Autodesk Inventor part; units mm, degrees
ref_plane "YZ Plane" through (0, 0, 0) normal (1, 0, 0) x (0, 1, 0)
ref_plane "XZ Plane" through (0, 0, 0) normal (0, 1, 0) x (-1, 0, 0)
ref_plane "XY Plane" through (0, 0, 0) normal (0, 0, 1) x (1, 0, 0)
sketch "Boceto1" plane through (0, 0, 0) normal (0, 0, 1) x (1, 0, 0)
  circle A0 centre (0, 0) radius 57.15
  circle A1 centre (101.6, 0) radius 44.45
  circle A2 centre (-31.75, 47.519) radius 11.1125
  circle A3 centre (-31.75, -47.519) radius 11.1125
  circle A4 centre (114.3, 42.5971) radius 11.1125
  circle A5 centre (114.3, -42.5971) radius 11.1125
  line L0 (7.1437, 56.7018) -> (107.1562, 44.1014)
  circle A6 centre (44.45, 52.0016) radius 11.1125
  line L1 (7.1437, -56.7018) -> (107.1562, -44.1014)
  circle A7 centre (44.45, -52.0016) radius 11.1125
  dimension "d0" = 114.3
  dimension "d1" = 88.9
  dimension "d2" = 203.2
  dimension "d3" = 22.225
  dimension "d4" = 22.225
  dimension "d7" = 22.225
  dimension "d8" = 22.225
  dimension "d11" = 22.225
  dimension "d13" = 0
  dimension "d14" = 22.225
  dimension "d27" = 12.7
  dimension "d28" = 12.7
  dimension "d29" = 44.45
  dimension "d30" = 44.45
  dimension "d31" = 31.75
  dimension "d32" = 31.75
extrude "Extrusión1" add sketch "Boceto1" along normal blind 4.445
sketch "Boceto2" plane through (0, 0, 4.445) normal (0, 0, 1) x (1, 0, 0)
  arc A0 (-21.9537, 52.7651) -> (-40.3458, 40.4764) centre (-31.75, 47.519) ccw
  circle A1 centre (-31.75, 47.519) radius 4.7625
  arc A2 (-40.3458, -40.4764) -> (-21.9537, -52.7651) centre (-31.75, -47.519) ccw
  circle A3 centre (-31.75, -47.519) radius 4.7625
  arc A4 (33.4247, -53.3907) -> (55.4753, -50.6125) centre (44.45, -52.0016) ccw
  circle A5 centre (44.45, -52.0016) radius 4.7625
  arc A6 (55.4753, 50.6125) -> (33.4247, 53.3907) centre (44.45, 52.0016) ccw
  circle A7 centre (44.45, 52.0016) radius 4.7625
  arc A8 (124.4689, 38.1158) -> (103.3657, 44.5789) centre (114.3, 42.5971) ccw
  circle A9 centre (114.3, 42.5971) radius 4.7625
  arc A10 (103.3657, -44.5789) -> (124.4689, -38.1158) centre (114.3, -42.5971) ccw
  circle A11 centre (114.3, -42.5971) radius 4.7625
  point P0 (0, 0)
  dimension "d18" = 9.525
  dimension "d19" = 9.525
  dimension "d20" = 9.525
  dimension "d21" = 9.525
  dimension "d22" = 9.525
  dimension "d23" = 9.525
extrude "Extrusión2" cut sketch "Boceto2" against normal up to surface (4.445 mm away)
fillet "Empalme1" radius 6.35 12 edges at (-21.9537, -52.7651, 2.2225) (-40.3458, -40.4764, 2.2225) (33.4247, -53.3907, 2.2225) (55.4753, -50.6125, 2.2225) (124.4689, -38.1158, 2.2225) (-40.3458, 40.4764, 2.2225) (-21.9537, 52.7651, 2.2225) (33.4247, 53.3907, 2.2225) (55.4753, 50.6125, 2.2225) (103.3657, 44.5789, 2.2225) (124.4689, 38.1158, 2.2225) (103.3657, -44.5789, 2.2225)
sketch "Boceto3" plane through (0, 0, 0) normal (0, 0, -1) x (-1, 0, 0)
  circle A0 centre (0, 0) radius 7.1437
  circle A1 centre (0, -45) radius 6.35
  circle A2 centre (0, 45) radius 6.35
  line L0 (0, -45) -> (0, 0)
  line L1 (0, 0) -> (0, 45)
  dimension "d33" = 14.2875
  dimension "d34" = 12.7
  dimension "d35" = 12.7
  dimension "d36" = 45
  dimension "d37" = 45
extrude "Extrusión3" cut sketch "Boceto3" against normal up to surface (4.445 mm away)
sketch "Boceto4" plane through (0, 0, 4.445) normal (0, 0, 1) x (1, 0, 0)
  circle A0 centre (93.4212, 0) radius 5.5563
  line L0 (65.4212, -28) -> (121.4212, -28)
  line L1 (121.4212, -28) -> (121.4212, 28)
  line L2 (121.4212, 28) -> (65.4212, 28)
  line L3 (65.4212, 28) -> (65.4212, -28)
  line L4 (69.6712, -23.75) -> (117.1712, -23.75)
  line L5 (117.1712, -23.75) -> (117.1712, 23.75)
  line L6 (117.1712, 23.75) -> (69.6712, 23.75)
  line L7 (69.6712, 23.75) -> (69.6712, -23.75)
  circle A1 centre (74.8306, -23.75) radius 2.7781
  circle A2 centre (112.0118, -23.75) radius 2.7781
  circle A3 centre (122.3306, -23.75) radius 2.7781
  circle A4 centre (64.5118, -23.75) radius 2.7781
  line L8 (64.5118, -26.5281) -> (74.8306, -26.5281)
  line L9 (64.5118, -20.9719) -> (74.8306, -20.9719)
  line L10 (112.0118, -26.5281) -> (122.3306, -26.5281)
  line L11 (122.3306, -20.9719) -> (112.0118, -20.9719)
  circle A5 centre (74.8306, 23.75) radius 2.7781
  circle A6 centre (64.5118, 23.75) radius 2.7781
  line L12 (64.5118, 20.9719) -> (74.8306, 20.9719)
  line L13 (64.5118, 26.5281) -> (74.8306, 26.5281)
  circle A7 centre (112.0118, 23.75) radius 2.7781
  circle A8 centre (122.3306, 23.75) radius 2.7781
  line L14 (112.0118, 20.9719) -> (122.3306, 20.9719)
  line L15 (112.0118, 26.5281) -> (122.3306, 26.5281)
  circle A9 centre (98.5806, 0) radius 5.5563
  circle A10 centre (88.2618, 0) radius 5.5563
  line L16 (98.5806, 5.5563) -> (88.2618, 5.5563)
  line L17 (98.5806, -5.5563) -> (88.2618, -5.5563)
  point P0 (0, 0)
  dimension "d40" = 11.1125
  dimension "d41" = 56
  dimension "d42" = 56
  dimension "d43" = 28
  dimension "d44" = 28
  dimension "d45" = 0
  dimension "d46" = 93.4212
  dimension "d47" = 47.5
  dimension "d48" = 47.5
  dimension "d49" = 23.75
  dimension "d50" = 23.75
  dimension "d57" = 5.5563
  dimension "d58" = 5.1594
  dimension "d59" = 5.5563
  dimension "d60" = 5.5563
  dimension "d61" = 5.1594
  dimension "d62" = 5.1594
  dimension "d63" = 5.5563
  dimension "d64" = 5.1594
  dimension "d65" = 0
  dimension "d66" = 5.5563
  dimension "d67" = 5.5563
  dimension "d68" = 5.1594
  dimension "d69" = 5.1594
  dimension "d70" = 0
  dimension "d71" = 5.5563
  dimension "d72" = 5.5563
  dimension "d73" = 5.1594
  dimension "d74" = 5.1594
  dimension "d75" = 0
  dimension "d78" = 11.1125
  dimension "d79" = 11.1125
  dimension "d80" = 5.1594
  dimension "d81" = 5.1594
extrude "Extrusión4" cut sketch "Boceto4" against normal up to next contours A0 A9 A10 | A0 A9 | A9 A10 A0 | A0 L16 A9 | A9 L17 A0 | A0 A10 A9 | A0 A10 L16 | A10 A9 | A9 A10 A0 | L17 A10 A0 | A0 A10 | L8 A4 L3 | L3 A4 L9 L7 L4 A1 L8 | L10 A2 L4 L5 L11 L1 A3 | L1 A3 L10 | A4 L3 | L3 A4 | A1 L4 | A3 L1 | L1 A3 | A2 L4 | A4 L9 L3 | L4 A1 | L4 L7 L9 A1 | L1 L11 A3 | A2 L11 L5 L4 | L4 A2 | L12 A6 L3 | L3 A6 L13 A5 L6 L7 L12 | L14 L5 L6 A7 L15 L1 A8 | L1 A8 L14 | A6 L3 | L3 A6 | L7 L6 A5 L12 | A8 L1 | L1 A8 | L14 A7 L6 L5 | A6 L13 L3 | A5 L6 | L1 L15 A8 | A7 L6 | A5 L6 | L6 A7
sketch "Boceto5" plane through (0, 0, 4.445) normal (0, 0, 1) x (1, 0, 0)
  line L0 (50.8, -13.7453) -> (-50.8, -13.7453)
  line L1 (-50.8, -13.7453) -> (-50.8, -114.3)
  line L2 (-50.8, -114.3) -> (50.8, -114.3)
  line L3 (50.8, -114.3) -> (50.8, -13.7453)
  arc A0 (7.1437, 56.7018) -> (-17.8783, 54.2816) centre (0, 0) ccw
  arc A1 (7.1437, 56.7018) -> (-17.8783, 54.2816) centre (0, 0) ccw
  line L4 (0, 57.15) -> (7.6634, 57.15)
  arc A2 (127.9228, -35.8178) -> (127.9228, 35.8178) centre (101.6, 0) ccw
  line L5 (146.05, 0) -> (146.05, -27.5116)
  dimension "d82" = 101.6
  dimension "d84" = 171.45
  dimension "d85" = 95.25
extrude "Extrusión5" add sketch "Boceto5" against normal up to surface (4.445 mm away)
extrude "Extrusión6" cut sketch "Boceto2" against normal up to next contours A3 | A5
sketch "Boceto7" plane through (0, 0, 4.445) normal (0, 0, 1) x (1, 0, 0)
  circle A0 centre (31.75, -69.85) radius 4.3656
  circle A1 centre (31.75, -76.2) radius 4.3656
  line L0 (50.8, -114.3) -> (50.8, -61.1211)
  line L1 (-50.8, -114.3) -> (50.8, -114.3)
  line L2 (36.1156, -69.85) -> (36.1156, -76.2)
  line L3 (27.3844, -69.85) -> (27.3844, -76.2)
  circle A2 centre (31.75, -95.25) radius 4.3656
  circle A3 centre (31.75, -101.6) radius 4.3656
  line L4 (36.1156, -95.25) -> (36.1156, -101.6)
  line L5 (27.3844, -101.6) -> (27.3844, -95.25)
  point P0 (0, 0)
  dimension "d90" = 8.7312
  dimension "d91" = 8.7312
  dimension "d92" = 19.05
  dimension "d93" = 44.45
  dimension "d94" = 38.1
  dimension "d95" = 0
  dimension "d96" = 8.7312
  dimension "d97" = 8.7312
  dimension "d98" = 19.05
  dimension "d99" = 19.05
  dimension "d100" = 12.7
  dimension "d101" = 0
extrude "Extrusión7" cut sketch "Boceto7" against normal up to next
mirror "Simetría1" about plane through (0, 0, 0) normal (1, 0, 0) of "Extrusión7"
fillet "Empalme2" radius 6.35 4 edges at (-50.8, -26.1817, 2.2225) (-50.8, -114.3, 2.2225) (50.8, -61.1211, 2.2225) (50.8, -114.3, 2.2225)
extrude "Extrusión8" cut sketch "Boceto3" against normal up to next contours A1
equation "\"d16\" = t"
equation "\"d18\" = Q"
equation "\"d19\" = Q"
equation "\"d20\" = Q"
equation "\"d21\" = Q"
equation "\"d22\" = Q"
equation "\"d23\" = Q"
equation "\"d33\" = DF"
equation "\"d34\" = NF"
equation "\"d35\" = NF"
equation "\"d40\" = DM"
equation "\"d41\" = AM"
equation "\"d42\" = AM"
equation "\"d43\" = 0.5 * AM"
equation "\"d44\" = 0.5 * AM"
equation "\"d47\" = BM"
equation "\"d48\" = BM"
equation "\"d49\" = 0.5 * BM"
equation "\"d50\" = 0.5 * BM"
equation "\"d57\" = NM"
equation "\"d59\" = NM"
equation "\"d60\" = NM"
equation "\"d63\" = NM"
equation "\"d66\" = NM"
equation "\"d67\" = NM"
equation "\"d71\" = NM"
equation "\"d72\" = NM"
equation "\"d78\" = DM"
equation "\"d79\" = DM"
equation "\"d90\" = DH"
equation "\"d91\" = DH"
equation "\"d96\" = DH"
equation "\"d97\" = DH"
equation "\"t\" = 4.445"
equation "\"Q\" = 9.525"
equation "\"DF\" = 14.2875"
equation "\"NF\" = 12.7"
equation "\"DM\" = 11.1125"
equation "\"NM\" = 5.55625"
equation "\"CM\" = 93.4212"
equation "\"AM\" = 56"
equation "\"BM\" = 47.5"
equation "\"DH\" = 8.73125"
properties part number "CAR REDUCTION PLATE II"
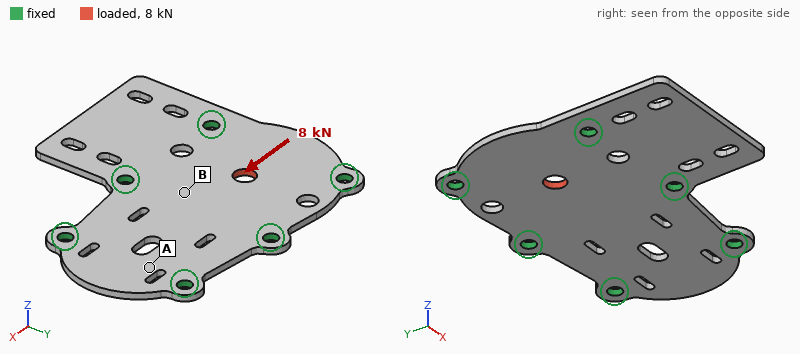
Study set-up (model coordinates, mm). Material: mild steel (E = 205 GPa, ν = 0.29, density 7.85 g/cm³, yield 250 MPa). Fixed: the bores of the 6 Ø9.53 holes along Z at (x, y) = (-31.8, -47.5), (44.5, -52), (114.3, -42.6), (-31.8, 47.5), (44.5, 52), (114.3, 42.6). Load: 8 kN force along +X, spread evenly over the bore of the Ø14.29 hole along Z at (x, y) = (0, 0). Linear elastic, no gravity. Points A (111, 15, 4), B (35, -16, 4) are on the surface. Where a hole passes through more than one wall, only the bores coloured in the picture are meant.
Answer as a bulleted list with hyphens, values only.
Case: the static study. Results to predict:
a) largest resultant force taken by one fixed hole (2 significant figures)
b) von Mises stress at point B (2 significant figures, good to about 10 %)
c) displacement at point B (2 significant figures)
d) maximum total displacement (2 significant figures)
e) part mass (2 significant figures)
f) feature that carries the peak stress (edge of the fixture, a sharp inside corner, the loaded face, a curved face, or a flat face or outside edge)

- 2.1 kN
- 12 MPa
- 2.9 µm
- 7.5 µm
- 840 g
- the loaded face
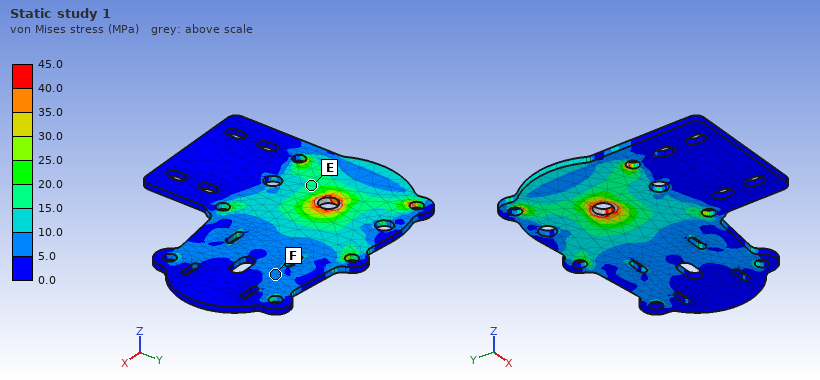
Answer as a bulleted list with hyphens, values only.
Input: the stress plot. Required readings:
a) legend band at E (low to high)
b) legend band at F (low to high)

- 15.0 to 20.0 MPa
- 5.0 to 10.0 MPa
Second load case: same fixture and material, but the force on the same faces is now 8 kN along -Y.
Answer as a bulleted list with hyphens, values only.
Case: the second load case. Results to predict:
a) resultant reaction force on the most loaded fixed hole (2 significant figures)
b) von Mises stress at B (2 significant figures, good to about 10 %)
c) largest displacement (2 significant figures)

- 2.5 kN
- 8.2 MPa
- 6.4 µm
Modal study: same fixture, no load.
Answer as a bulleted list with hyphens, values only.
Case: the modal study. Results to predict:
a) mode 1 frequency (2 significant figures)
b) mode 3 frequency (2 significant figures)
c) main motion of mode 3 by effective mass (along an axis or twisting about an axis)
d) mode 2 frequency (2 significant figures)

- 840 Hz
- 2100 Hz
- along Z
- 1700 Hz
